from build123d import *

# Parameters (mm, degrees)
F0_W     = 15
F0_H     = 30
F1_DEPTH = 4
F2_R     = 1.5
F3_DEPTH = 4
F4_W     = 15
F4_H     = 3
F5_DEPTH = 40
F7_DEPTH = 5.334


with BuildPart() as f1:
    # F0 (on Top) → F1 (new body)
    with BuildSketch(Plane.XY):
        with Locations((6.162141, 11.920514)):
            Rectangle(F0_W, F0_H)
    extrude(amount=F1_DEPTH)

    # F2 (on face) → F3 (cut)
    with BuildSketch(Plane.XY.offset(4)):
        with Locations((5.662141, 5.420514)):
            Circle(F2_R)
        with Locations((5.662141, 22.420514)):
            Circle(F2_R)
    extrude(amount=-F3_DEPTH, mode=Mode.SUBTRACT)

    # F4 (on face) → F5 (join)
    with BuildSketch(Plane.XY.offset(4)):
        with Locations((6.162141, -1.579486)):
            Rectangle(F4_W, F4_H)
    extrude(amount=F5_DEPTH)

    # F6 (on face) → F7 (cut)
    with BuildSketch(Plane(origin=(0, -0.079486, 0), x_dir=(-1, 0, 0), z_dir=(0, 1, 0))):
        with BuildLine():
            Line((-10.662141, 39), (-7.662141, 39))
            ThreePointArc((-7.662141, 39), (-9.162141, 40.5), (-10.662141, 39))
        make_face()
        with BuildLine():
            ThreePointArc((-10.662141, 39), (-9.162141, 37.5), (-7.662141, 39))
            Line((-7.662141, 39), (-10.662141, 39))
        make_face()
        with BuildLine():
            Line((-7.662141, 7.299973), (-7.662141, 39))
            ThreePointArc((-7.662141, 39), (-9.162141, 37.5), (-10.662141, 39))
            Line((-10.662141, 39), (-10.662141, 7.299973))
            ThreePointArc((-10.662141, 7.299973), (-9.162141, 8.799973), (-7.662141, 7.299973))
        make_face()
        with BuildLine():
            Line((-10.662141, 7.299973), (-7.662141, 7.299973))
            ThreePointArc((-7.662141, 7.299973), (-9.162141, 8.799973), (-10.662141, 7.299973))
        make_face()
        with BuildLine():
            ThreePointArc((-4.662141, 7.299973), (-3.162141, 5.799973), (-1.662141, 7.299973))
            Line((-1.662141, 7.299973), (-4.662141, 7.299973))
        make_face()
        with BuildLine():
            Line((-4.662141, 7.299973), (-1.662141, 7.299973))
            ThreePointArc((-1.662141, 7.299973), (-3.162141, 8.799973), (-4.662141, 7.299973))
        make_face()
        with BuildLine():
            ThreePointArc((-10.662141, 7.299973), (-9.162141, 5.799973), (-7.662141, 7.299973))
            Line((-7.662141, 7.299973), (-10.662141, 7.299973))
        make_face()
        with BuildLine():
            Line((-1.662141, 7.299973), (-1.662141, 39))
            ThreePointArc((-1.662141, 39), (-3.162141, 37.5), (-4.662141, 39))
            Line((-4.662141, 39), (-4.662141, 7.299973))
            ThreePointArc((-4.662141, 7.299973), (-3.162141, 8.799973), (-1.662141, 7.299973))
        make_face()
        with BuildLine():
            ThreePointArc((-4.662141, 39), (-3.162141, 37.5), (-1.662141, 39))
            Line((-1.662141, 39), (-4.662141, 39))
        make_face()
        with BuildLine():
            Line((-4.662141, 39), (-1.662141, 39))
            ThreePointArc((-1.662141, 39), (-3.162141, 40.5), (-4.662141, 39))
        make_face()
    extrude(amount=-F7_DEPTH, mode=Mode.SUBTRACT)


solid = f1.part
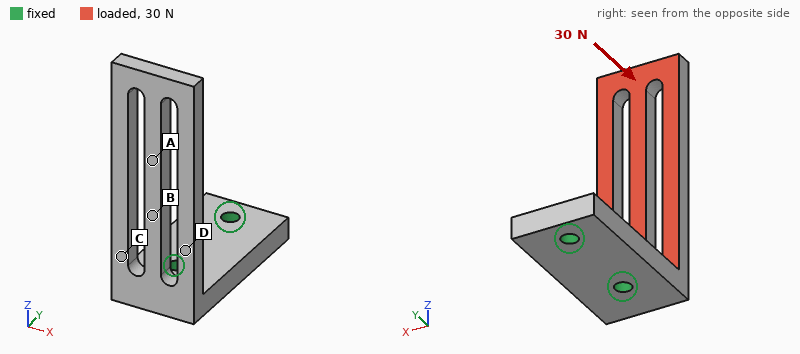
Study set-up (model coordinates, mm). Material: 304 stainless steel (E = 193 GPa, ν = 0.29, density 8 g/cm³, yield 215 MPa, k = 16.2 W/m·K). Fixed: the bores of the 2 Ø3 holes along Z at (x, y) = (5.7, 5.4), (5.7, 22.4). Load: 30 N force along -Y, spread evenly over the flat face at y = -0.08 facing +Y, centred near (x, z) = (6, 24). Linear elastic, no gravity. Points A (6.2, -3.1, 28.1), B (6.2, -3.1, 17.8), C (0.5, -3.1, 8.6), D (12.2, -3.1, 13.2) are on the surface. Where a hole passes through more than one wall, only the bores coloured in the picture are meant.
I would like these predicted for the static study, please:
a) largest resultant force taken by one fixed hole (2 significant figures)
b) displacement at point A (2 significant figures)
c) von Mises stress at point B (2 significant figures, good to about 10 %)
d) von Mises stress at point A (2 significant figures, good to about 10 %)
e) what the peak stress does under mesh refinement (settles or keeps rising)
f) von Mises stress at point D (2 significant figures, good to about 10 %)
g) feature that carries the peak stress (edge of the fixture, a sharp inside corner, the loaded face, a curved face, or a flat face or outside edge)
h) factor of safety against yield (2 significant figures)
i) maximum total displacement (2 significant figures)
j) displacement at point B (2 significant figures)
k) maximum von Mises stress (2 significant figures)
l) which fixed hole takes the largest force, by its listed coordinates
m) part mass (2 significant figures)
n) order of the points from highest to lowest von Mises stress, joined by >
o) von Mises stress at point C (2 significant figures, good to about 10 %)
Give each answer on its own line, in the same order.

29 N
39 µm
21 MPa
8.3 MPa
settles
27 MPa
the loaded face
4.2
78 µm
17 µm
52 MPa
(5.7, 5.4)
23 g
C > D > B > A
35 MPa
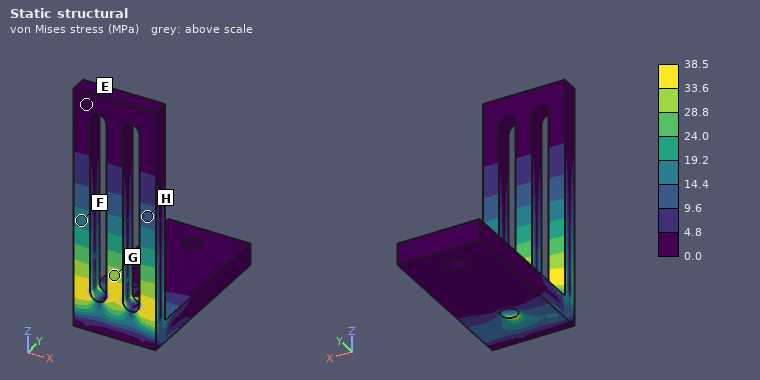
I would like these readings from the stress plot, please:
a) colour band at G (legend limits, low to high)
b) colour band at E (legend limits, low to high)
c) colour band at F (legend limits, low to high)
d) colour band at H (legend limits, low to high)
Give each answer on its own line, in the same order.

28.8 to 33.6 MPa
0.0 to 4.8 MPa
14.4 to 19.2 MPa
9.6 to 14.4 MPa
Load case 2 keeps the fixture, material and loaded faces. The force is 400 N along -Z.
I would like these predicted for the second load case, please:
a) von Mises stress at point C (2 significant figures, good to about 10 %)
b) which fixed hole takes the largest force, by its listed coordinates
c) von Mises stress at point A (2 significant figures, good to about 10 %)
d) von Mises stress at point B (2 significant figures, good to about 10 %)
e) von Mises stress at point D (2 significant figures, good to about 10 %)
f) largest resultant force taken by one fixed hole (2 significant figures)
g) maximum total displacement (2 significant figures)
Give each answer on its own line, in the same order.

25 MPa
(5.7, 5.4)
11 MPa
19 MPa
23 MPa
430 N
65 µm
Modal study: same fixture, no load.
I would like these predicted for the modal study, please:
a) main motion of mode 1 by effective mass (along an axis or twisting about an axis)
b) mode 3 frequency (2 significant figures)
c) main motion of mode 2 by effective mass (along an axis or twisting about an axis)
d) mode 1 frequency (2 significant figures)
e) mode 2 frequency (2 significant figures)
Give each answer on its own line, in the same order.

along Y
4600 Hz
along X
1200 Hz
2000 Hz
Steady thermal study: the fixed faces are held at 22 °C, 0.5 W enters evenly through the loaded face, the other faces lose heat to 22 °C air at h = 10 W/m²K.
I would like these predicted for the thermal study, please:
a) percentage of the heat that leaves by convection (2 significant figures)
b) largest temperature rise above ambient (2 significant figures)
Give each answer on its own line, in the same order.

30 %
18 K
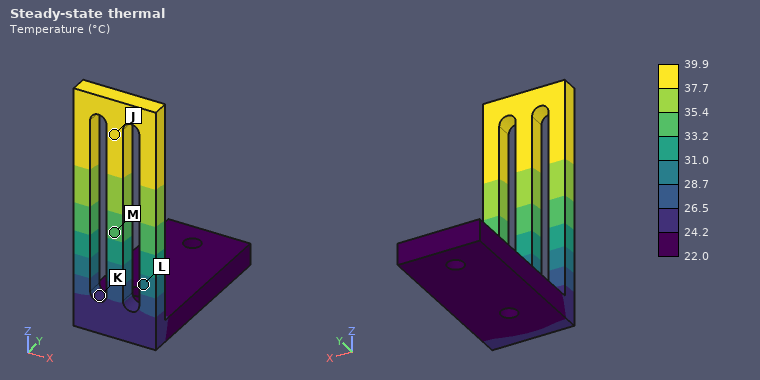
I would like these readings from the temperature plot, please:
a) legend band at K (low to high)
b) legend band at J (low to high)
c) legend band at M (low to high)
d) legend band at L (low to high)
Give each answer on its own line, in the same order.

24.2 to 26.5 °C
37.7 to 39.9 °C
33.2 to 35.4 °C
28.7 to 31.0 °C
